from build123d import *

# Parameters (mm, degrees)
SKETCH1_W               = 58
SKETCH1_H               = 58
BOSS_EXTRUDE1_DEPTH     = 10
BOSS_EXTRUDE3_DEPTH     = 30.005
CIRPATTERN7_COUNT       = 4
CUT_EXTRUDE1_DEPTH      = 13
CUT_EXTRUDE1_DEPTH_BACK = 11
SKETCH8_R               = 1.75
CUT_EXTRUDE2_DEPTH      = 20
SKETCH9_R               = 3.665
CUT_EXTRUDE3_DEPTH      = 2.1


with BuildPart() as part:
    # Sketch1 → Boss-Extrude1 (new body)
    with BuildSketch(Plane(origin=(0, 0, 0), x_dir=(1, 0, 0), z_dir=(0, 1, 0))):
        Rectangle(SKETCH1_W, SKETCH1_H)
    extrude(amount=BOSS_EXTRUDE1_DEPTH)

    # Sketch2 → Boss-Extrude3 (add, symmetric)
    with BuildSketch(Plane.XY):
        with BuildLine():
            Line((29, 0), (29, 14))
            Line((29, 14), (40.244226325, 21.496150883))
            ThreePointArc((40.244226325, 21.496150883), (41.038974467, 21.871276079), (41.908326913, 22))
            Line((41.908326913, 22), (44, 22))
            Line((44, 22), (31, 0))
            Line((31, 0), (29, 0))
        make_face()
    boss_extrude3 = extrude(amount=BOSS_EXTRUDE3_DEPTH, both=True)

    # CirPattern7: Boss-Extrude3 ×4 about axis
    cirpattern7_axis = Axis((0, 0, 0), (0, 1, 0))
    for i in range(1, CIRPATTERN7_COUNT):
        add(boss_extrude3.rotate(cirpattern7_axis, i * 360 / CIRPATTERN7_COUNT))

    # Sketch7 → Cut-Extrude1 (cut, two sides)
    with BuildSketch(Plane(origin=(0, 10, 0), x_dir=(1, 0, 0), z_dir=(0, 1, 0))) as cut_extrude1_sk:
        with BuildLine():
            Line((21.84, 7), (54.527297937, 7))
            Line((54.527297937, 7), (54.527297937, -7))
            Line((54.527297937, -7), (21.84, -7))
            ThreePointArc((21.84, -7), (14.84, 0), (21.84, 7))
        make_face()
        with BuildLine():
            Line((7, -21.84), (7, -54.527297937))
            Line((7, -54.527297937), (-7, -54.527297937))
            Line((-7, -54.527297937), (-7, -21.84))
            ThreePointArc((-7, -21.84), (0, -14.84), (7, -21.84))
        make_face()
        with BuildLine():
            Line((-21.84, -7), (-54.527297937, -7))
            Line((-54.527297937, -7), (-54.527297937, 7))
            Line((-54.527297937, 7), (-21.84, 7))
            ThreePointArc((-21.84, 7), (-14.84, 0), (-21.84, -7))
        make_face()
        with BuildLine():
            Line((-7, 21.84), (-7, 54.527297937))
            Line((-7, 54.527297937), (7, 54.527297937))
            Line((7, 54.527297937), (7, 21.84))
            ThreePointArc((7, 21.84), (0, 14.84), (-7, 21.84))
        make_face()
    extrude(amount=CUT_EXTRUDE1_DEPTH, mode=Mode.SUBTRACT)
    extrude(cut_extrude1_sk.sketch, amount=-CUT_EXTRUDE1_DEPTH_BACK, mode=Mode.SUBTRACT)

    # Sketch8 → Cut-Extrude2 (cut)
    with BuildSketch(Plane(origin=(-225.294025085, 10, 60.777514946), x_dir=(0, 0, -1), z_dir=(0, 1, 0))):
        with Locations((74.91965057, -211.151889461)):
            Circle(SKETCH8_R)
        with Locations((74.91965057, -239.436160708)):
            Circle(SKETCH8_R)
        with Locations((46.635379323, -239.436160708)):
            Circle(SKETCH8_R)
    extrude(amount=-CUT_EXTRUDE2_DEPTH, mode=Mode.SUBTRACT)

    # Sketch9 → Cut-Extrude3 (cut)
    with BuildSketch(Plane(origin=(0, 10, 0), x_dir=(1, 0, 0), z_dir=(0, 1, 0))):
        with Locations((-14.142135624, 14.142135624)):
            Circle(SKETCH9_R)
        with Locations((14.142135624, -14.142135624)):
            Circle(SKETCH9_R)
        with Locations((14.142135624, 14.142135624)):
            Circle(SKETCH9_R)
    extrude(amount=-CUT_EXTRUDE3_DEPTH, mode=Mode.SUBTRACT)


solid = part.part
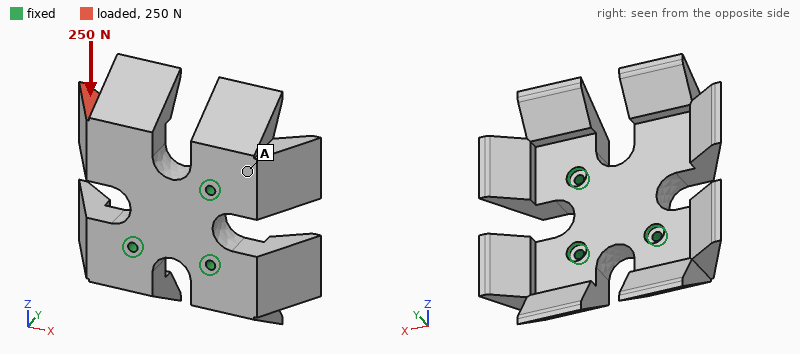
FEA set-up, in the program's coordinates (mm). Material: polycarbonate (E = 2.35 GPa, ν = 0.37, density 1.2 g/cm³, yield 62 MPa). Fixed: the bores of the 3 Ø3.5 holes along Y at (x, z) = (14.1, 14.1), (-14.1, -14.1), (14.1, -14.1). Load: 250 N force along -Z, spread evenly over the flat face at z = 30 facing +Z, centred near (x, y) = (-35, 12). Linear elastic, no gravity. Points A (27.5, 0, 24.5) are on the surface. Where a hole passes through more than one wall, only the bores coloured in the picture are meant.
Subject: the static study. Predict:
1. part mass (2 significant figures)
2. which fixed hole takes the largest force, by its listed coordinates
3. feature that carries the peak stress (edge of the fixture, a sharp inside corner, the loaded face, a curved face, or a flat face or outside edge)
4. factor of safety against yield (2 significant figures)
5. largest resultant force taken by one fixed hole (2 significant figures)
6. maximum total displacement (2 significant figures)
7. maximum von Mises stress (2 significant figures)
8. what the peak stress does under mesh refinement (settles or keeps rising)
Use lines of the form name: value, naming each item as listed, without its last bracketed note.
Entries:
part mass: 62 g
which fixed hole takes the largest force, by its listed coordinates: (-14.1, -14.1)
feature that carries the peak stress: a curved face
factor of safety against yield: 2.5
largest resultant force taken by one fixed hole: 270 N
maximum total displacement: 0.81 mm
maximum von Mises stress: 25 MPa
what the peak stress does under mesh refinement: settles
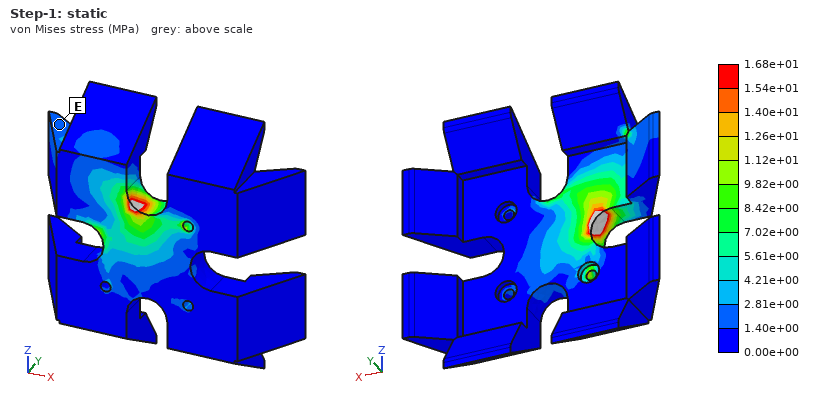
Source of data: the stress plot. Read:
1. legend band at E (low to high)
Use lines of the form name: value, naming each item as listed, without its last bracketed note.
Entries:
legend band at E: 1.40e+00 to 2.81e+00 MPa
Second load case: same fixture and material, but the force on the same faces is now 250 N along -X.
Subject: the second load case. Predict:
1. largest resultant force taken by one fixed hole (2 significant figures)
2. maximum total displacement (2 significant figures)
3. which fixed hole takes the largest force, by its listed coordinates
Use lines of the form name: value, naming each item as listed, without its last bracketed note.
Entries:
largest resultant force taken by one fixed hole: 240 N
maximum total displacement: 0.94 mm
which fixed hole takes the largest force, by its listed coordinates: (14.1, 14.1)
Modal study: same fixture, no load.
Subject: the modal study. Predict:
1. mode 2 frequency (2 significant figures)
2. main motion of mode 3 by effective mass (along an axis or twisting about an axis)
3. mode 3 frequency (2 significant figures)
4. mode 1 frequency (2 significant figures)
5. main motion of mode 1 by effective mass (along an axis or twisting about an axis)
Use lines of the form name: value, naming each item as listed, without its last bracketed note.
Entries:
mode 2 frequency: 1200 Hz
main motion of mode 3 by effective mass: along Y
mode 3 frequency: 1500 Hz
mode 1 frequency: 610 Hz
main motion of mode 1 by effective mass: along Y
